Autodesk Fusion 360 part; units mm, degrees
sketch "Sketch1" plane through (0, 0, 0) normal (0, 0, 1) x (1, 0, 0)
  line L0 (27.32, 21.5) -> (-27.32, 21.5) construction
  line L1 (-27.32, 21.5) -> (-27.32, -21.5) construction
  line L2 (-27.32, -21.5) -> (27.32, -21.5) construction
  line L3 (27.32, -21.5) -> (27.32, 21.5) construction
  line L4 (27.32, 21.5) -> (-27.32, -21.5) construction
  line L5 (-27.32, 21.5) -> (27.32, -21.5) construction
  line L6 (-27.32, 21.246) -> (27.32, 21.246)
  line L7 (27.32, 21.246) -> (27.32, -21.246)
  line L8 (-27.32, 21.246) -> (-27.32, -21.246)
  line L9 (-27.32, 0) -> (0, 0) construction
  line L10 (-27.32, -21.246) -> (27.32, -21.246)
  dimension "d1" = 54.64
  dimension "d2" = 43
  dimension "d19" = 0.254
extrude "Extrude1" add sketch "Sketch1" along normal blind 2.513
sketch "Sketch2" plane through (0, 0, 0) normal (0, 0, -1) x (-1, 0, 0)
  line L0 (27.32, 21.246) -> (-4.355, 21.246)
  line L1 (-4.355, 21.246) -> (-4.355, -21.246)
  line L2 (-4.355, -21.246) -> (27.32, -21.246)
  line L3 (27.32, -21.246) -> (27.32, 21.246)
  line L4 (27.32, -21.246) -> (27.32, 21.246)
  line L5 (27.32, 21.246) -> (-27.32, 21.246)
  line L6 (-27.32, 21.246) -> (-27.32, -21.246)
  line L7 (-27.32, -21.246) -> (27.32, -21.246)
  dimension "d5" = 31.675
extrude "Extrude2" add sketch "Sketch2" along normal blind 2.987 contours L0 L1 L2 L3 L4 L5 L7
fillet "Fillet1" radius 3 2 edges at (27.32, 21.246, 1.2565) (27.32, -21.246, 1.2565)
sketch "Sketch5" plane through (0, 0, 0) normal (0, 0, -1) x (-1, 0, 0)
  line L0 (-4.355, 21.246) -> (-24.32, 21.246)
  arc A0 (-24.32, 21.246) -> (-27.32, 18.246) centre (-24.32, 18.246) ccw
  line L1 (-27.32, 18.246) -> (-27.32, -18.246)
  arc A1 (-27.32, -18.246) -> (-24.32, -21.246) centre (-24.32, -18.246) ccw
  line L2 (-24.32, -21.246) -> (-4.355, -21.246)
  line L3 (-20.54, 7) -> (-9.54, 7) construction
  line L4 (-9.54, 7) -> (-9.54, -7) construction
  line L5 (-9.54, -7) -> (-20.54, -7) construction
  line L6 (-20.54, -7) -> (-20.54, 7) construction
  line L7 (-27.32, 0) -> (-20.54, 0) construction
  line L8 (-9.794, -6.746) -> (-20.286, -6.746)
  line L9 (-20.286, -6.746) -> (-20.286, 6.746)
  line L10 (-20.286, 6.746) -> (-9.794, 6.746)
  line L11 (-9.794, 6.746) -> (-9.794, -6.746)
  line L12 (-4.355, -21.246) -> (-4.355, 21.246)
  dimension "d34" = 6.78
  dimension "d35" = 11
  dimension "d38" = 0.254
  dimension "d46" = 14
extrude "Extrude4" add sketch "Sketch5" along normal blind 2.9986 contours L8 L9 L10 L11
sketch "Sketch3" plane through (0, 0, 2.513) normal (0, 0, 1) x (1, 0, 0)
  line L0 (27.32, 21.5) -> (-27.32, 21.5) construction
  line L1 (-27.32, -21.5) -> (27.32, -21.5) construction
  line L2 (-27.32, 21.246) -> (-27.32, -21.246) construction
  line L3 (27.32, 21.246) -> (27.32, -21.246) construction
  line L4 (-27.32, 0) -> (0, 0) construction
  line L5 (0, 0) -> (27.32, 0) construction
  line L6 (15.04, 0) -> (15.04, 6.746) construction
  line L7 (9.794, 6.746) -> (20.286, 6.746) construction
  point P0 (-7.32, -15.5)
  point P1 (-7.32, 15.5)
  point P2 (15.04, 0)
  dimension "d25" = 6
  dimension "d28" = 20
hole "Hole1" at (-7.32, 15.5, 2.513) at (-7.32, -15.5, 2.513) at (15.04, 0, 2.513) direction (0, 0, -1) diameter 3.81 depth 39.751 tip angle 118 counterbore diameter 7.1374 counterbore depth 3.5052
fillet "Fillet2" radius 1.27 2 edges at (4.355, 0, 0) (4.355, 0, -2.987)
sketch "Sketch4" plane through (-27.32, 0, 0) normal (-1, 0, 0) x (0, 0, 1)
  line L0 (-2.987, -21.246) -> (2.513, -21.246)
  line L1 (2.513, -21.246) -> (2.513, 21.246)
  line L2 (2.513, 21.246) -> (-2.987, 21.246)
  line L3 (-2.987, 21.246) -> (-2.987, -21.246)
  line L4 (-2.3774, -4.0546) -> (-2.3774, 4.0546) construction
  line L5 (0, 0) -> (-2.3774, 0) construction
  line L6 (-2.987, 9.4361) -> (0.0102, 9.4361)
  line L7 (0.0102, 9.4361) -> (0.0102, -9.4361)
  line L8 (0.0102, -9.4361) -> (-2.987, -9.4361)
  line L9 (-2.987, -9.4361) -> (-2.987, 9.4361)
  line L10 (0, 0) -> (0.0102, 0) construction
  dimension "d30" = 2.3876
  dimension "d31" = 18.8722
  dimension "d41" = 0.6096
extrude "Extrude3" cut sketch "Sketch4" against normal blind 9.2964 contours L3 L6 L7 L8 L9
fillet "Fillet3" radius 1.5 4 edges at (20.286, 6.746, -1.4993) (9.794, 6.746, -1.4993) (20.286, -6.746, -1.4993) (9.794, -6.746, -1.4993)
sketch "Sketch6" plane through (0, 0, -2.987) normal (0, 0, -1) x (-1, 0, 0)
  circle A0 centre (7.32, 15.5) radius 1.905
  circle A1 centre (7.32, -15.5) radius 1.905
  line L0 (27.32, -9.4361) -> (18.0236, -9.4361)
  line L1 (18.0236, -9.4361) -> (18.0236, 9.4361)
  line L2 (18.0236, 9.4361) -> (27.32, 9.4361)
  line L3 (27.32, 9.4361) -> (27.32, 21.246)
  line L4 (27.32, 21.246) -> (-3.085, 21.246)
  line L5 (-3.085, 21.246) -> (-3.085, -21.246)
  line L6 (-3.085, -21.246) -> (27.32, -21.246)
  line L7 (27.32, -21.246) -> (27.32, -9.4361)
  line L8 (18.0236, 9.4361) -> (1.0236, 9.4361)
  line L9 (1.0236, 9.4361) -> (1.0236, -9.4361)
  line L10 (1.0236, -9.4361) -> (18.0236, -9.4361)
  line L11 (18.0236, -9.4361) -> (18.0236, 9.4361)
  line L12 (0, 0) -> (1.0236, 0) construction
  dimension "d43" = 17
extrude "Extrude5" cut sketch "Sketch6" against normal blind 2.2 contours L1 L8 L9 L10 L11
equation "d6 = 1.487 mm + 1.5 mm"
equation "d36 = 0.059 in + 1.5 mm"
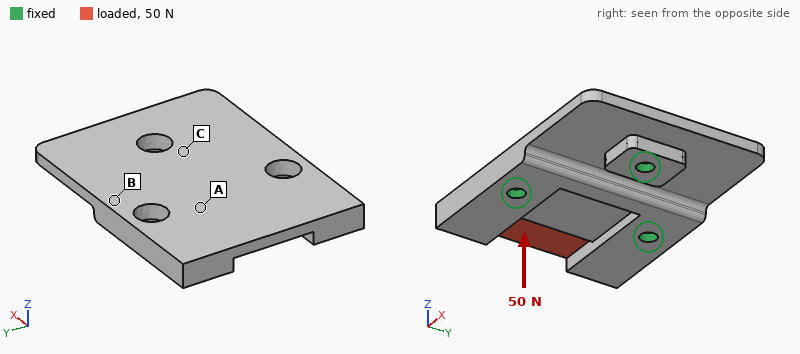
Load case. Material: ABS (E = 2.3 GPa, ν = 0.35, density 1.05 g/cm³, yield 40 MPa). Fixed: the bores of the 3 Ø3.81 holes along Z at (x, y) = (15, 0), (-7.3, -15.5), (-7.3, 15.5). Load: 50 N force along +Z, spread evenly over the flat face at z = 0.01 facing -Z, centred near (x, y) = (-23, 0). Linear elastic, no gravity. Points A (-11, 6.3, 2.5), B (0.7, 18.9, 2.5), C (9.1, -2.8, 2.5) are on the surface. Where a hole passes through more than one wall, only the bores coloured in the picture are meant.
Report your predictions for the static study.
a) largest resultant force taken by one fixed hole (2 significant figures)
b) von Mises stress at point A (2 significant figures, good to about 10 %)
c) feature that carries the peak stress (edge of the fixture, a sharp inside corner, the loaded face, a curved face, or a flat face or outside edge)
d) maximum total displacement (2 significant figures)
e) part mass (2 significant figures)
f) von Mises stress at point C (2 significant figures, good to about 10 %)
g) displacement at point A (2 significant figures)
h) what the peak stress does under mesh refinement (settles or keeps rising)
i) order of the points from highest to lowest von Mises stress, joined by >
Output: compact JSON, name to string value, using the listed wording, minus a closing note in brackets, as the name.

{"largest resultant force taken by one fixed hole": "65 N", "von Mises stress at point A": "4.2 MPa", "feature that carries the peak stress": "edge of the fixture", "maximum total displacement": "0.30 mm", "part mass": "9.0 g", "von Mises stress at point C": "1.7 MPa", "displacement at point A": "0.059 mm", "what the peak stress does under mesh refinement": "keeps rising", "order of the points from highest to lowest von Mises stress, joined by >": "A > C > B"}
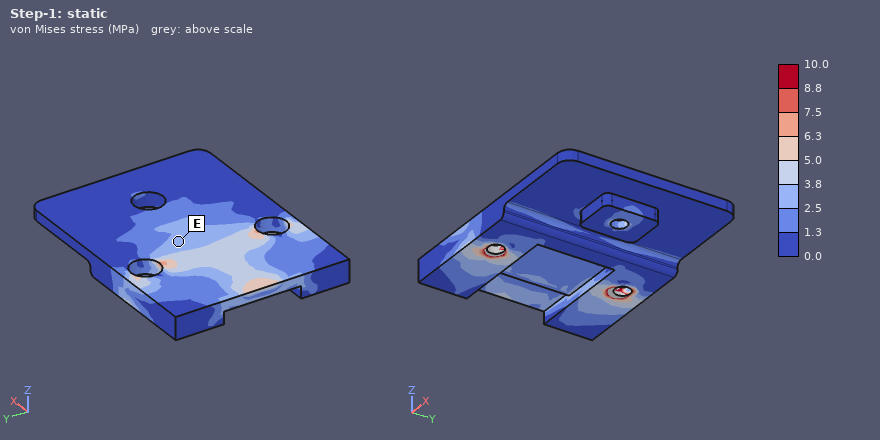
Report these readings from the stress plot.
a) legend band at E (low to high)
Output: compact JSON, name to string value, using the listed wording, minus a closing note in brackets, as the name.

{"legend band at E": "2.5 to 3.8 MPa"}
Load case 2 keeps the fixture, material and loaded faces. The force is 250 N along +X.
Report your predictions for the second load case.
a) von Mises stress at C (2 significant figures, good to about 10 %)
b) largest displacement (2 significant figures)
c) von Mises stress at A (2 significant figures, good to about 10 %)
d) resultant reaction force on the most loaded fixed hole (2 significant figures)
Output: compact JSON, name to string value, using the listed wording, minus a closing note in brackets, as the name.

{"von Mises stress at C": "1.9 MPa", "largest displacement": "64 µm", "von Mises stress at A": "3.0 MPa", "resultant reaction force on the most loaded fixed hole": "100 N"}
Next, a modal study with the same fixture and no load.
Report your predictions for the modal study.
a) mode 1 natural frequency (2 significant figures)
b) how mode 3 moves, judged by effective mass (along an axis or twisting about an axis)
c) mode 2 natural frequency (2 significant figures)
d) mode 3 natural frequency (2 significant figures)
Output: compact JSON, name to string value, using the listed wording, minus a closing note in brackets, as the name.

{"mode 1 natural frequency": "2000 Hz", "how mode 3 moves, judged by effective mass": "along Z", "mode 2 natural frequency": "2200 Hz", "mode 3 natural frequency": "2600 Hz"}
